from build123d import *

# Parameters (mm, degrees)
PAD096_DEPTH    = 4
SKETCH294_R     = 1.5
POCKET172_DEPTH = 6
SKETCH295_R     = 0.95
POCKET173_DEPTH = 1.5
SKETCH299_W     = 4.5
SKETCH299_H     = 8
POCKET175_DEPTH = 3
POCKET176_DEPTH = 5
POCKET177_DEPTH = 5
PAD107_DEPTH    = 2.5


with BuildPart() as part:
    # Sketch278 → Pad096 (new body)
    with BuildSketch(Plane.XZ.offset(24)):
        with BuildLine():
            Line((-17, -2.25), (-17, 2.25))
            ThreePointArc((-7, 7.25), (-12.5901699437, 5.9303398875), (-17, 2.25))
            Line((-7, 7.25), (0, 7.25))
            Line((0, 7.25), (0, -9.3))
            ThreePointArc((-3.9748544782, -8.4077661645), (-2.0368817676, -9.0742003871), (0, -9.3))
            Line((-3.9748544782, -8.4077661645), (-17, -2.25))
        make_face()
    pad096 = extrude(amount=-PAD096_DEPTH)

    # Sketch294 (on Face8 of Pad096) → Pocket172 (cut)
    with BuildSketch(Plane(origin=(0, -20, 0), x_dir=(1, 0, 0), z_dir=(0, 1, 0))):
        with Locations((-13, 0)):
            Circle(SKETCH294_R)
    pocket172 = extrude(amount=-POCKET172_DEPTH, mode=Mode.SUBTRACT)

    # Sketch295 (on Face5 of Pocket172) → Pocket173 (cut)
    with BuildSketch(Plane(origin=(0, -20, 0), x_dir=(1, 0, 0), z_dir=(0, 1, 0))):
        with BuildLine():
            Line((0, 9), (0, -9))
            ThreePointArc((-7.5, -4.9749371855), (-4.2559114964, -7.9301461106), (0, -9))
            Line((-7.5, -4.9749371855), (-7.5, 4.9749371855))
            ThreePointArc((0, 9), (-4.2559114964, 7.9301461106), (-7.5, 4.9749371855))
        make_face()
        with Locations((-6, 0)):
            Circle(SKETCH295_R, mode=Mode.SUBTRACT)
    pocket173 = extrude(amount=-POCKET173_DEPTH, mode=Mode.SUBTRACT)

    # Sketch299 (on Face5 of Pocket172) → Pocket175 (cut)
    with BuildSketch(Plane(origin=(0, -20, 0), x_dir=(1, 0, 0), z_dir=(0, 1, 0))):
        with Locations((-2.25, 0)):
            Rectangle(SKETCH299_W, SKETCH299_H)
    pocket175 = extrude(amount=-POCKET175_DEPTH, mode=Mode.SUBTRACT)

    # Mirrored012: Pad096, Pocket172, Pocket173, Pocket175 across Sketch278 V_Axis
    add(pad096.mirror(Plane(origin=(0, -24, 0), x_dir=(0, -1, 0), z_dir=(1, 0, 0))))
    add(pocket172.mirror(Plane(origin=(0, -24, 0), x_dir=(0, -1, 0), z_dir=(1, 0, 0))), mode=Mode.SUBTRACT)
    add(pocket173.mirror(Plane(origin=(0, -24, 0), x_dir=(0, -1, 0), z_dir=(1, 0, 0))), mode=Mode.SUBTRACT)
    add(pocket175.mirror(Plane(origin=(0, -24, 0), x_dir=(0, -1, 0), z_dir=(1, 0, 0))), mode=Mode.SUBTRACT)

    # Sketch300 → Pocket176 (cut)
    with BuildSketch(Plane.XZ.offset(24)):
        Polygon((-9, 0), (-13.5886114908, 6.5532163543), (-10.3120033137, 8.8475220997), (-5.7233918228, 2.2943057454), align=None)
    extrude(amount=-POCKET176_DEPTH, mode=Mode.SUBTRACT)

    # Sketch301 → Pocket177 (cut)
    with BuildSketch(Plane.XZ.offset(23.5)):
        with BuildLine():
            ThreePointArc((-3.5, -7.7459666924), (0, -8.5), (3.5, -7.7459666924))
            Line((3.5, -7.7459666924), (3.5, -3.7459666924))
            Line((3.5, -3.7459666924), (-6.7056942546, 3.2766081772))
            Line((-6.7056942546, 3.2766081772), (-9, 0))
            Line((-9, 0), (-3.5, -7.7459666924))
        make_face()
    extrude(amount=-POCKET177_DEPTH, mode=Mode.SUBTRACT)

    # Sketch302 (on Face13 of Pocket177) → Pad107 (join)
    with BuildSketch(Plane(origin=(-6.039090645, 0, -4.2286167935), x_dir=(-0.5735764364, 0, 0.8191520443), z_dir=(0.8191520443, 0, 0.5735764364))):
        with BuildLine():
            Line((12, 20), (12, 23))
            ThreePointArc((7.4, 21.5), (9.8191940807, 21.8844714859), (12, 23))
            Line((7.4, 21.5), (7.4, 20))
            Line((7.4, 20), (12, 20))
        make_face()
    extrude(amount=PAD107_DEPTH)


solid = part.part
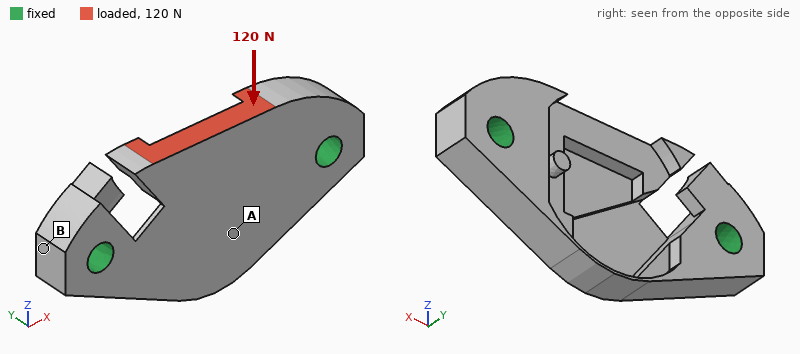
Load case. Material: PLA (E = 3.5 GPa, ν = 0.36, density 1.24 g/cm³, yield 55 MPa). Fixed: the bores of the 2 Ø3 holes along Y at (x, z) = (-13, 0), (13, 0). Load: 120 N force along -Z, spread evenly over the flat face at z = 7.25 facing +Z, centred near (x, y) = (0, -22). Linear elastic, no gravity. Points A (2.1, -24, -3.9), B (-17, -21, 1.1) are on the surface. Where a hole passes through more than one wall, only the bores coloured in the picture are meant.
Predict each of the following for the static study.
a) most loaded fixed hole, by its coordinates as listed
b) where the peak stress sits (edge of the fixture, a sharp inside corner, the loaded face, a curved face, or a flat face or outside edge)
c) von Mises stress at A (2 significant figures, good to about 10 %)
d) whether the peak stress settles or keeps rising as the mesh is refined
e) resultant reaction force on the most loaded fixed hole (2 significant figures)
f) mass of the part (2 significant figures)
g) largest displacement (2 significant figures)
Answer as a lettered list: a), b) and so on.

a) (13, 0)
b) a sharp inside corner
c) 8.8 MPa
d) keeps rising
e) 71 N
f) 1.3 g
g) 0.36 mm
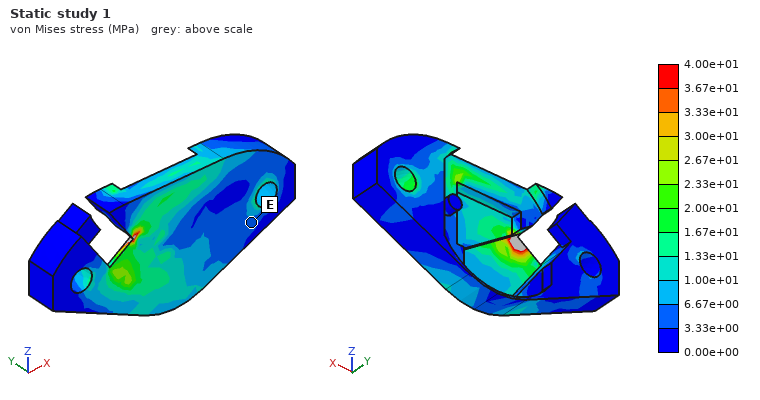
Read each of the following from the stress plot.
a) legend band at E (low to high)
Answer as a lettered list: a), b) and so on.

a) 3.33e+00 to 6.67e+00 MPa
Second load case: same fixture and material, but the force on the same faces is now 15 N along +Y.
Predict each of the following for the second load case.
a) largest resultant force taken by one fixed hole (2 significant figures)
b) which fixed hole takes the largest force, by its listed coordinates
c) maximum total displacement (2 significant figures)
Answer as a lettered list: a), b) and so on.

a) 15 N
b) (13, 0)
c) 0.38 mm
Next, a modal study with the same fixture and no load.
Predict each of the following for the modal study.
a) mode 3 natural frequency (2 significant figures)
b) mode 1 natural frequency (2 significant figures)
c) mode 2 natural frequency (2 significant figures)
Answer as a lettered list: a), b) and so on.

a) 8900 Hz
b) 3000 Hz
c) 8500 Hz
